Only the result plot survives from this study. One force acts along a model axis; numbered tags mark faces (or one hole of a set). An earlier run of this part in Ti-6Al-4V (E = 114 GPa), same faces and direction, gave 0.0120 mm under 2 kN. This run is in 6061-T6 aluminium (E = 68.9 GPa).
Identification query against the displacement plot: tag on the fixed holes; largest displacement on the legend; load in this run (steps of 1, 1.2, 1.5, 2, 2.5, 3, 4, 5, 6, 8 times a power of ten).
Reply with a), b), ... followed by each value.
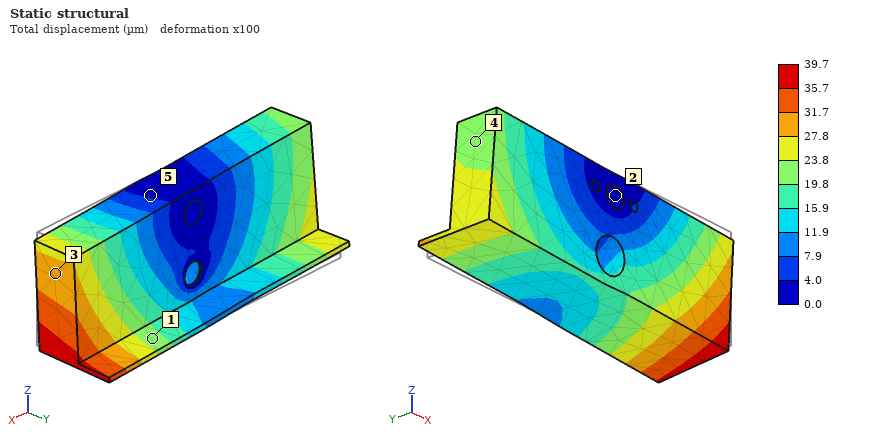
a) 2
b) 39.7 µm
c) 4 kN
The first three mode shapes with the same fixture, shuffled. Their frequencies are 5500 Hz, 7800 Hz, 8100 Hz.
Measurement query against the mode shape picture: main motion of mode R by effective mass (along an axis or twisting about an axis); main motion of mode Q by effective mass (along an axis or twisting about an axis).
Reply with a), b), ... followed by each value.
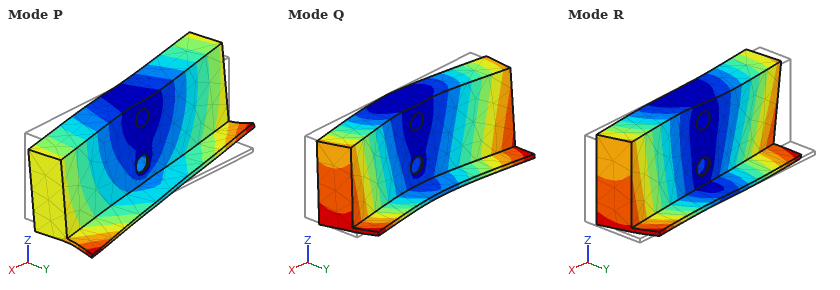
a) twisting about Z
b) along Y
